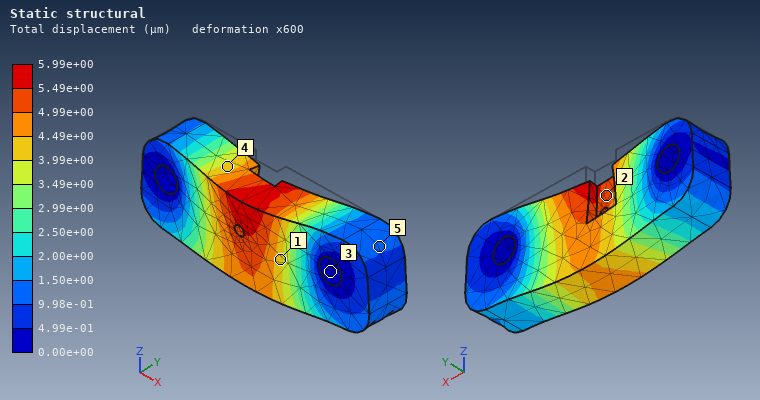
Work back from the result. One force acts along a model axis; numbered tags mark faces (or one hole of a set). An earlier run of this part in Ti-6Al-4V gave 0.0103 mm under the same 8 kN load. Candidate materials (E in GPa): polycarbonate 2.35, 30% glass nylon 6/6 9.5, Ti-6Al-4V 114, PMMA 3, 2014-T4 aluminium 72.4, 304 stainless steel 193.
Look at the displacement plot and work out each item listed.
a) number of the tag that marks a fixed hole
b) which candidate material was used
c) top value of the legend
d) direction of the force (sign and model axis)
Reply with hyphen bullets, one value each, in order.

- 3
- 304 stainless steel
- 5.99e+00 µm
- -Z
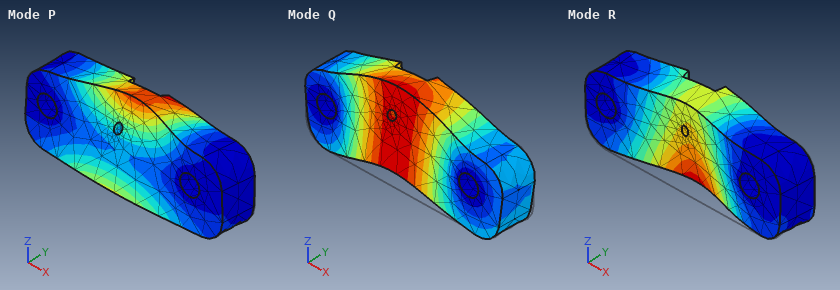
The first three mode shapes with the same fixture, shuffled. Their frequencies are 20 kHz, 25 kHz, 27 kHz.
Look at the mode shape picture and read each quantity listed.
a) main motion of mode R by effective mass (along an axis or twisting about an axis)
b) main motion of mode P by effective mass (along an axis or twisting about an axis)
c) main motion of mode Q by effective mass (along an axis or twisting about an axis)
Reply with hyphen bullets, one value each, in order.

- along Y
- twisting about X
- along Z
